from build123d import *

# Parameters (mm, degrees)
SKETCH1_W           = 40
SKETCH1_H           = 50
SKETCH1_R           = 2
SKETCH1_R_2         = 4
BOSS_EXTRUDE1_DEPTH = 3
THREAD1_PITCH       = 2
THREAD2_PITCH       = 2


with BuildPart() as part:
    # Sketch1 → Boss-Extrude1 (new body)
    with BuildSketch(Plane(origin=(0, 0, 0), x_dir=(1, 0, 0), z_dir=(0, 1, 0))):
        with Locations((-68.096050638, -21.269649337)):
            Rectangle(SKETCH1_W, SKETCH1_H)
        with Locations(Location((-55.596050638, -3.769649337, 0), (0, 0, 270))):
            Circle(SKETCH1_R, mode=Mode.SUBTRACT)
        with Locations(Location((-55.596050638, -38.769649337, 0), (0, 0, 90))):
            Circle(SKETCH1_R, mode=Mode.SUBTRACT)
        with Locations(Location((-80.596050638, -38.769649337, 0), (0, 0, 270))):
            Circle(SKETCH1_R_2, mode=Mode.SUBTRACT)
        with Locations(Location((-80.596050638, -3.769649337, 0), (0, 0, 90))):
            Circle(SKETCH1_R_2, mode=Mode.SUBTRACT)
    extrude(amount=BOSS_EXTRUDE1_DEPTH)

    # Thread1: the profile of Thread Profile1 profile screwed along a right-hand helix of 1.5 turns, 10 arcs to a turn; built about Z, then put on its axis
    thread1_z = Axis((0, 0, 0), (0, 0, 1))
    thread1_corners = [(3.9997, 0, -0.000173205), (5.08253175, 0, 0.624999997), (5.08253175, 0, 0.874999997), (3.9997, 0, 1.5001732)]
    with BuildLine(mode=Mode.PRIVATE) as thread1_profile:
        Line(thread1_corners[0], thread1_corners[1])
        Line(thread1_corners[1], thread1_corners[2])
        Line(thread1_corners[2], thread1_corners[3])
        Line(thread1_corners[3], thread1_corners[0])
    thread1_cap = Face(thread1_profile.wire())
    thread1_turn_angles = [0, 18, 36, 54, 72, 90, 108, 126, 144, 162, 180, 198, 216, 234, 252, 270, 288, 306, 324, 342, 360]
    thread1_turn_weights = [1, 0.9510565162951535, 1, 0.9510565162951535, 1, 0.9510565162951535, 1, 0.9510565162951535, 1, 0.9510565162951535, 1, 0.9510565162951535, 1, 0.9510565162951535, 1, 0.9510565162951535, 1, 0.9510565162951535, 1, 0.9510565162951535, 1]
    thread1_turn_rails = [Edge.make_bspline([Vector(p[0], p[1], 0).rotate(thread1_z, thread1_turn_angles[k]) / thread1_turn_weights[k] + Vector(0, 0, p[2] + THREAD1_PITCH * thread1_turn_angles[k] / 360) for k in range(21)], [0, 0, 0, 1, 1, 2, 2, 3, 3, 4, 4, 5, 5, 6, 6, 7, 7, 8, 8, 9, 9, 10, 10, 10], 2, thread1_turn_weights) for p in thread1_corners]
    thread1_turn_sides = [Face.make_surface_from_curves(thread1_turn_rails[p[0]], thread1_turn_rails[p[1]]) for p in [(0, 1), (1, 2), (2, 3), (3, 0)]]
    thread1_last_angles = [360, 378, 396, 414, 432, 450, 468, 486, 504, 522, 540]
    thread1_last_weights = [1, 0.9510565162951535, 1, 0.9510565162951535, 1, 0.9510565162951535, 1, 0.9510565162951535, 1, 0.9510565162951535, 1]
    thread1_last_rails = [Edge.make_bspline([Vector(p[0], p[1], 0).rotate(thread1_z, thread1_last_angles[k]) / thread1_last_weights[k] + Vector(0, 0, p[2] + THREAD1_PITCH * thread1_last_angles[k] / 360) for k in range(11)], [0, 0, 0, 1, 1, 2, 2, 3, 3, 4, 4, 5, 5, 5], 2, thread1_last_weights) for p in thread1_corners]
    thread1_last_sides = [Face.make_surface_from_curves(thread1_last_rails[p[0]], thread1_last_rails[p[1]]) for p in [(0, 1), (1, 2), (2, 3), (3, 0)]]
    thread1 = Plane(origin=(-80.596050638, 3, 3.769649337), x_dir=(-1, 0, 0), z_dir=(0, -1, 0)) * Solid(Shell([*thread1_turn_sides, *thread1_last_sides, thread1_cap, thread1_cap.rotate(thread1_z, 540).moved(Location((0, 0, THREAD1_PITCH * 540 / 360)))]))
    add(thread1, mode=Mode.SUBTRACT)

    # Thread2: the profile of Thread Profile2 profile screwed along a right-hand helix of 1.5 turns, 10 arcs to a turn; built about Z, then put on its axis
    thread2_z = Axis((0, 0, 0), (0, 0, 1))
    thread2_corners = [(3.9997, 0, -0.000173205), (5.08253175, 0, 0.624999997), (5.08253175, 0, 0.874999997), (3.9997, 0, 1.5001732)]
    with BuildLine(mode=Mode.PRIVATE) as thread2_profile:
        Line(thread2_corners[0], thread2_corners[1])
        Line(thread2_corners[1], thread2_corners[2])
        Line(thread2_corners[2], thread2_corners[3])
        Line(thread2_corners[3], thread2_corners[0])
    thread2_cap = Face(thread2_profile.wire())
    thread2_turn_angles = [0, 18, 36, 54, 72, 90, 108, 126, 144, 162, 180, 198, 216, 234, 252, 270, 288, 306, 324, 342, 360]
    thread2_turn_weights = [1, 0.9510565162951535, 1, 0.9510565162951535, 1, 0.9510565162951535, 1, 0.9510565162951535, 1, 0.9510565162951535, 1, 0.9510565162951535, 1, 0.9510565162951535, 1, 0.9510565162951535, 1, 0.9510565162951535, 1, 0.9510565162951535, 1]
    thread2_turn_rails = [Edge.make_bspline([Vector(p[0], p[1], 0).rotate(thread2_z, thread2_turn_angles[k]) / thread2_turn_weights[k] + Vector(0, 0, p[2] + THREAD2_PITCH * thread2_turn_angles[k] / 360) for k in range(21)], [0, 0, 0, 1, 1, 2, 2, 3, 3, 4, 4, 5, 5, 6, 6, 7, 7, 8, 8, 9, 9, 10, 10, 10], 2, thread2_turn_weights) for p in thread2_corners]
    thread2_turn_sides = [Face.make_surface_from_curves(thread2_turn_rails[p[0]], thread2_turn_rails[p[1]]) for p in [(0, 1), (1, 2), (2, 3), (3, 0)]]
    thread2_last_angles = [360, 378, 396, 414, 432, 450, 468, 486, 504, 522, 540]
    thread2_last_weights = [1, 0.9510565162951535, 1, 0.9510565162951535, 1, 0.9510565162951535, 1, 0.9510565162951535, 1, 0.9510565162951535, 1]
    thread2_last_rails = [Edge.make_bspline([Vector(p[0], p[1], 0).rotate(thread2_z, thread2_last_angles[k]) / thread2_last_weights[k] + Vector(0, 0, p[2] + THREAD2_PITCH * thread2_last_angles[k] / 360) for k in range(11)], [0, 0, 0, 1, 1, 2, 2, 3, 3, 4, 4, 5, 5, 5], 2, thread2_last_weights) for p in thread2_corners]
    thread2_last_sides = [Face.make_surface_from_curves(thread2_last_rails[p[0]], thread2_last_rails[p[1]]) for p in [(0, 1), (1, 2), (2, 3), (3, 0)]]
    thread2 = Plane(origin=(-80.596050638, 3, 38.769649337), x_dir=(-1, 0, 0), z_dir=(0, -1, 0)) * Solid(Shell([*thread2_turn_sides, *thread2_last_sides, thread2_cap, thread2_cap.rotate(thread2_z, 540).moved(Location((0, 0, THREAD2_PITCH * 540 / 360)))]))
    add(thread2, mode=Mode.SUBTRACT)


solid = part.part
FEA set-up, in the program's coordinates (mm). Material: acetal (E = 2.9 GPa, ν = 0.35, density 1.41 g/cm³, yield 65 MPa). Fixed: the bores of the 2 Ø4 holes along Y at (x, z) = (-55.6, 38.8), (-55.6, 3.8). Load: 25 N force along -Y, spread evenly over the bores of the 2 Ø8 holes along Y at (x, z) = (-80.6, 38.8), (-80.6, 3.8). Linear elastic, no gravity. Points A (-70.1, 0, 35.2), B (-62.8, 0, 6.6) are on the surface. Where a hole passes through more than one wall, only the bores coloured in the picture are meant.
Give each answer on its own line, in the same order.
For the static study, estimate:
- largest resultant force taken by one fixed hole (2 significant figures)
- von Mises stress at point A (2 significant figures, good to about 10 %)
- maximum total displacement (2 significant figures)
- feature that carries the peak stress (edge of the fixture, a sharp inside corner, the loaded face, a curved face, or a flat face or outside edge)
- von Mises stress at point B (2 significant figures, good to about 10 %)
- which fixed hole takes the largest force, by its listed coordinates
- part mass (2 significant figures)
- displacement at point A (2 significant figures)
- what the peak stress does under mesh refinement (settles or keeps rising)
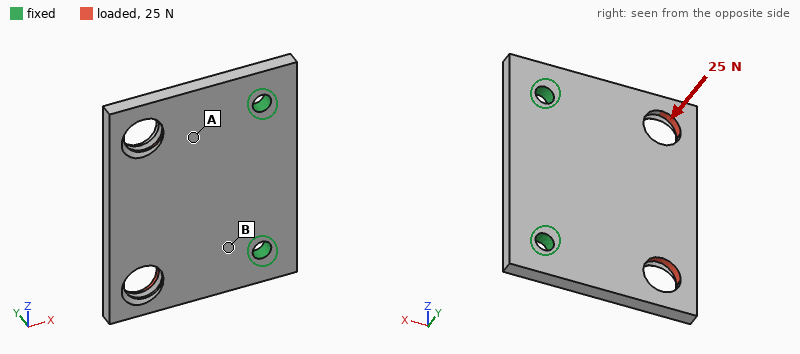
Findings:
14 N
3.2 MPa
0.69 mm
edge of the fixture
6.5 MPa
(-55.6, 3.8)
7.8 g
0.19 mm
keeps rising
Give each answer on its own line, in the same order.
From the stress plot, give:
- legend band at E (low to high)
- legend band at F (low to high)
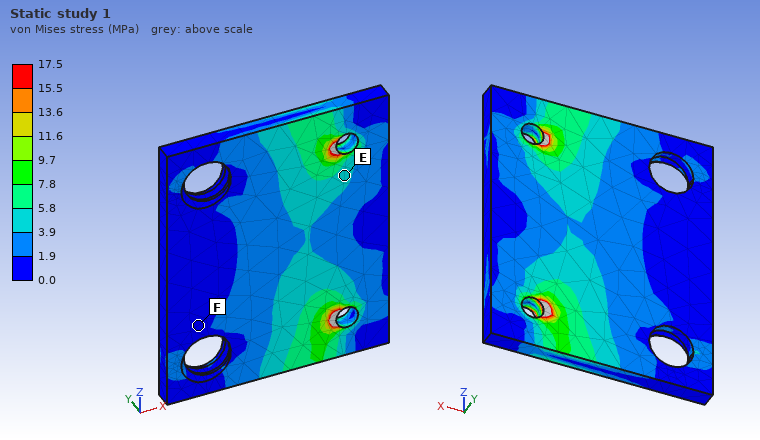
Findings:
3.9 to 5.8 MPa
0.0 to 1.9 MPa
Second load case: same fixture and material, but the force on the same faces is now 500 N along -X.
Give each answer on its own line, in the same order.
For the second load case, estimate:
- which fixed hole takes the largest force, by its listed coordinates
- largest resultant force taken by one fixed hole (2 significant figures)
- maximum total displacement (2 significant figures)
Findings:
(-55.6, 3.8)
280 N
0.42 mm
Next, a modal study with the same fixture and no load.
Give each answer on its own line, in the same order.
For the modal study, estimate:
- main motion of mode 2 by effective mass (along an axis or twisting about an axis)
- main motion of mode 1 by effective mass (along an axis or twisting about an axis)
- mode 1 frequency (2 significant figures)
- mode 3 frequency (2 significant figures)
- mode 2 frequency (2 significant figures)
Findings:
twisting about X
along Y
660 Hz
2500 Hz
1300 Hz
